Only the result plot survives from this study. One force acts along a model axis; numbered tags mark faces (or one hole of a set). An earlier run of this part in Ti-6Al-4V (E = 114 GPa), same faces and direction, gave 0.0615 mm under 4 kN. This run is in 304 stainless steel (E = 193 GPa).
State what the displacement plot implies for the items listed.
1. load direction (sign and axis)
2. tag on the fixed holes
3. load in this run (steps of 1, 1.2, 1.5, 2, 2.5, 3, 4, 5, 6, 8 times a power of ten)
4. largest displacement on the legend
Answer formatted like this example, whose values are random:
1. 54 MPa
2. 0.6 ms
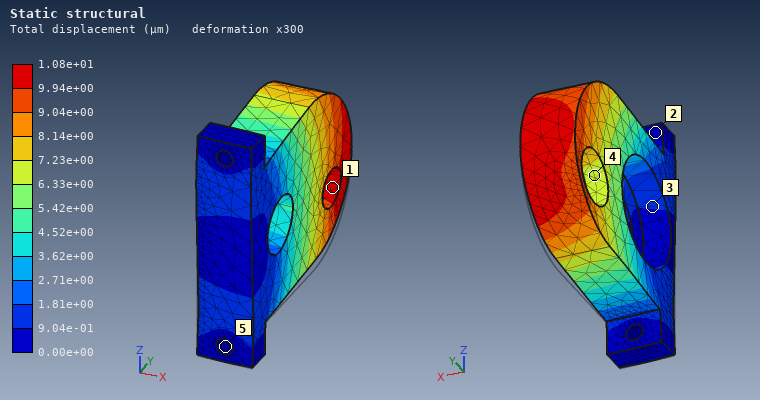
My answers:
1. +Z
2. 5
3. 1.2 kN
4. 1.08e+01 µm
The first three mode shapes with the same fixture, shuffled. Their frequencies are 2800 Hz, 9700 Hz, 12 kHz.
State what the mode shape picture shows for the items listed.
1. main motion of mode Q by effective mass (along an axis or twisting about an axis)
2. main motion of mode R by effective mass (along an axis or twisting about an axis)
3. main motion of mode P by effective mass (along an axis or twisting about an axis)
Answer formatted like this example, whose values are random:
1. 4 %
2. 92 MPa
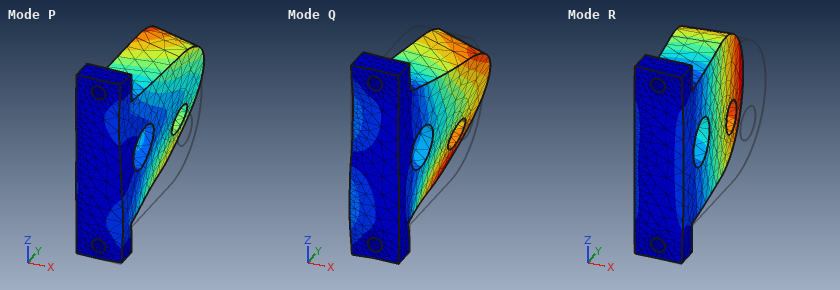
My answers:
1. along Z
2. along X
3. along Z
